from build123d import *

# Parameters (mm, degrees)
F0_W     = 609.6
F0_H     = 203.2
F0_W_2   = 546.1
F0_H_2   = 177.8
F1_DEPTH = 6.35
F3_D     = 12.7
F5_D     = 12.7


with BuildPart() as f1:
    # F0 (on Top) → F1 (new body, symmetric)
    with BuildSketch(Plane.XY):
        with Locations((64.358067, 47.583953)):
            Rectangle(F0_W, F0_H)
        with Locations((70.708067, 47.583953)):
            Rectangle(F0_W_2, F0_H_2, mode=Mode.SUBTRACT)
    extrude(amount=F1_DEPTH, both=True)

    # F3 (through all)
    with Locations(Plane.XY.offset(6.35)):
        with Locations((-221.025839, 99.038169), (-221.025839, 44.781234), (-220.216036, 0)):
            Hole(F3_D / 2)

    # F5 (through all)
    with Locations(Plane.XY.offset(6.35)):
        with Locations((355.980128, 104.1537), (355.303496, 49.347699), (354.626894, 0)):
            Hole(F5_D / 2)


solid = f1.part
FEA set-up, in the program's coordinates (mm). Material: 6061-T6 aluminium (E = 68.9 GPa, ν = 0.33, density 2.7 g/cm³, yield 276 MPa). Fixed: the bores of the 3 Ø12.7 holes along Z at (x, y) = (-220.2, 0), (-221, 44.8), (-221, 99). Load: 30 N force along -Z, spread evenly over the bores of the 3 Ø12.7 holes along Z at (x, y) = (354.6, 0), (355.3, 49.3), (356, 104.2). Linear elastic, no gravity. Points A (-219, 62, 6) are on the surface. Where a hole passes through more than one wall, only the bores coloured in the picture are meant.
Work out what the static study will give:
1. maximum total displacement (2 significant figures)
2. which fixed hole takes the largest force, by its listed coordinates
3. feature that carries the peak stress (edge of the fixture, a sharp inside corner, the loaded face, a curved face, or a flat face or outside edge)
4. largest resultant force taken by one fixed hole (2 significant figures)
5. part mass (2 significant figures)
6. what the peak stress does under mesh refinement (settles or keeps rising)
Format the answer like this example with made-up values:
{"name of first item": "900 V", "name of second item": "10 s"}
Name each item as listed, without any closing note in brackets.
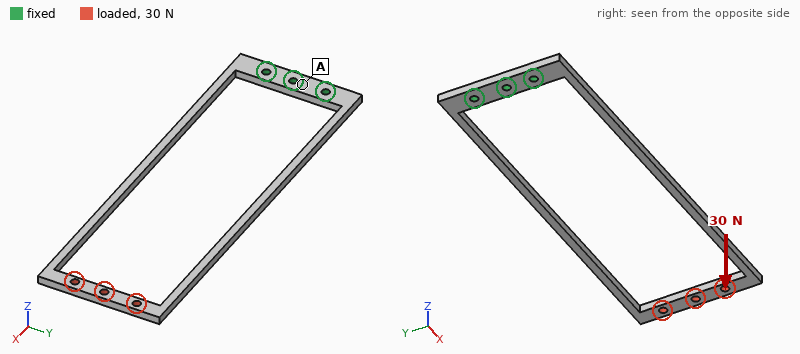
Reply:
{"maximum total displacement": "6.7 mm", "which fixed hole takes the largest force, by its listed coordinates": "(-221, 99)", "feature that carries the peak stress": "a sharp inside corner", "largest resultant force taken by one fixed hole": "16 N", "part mass": "890 g", "what the peak stress does under mesh refinement": "keeps rising"}
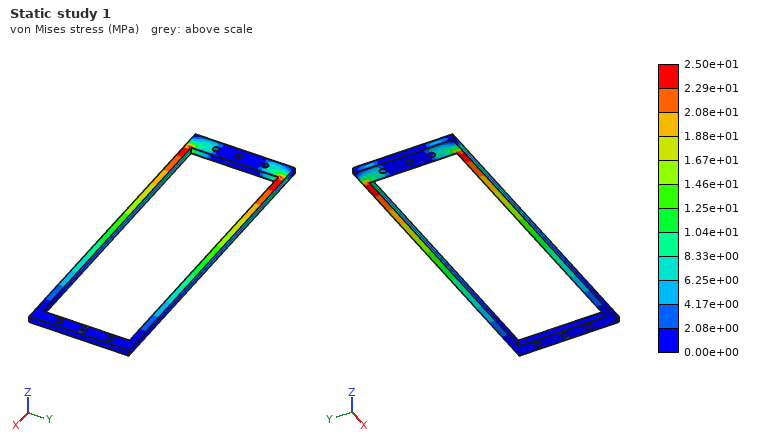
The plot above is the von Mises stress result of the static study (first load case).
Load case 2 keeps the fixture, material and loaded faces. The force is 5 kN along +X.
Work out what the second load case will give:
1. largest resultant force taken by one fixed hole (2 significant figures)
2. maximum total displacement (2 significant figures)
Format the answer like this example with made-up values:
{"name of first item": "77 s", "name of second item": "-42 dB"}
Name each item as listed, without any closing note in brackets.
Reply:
{"largest resultant force taken by one fixed hole": "3.6 kN", "maximum total displacement": "0.74 mm"}
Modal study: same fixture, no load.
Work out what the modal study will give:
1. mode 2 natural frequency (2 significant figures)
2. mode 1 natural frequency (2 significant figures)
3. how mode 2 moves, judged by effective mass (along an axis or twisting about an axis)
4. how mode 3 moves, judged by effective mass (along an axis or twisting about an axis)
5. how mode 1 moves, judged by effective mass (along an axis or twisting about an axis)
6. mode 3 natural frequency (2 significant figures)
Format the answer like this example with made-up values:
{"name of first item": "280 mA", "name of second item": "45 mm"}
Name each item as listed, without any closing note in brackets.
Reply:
{"mode 2 natural frequency": "38 Hz", "mode 1 natural frequency": "21 Hz", "how mode 2 moves, judged by effective mass": "along Y", "how mode 3 moves, judged by effective mass": "twisting about X", "how mode 1 moves, judged by effective mass": "along Z", "mode 3 natural frequency": "74 Hz"}
